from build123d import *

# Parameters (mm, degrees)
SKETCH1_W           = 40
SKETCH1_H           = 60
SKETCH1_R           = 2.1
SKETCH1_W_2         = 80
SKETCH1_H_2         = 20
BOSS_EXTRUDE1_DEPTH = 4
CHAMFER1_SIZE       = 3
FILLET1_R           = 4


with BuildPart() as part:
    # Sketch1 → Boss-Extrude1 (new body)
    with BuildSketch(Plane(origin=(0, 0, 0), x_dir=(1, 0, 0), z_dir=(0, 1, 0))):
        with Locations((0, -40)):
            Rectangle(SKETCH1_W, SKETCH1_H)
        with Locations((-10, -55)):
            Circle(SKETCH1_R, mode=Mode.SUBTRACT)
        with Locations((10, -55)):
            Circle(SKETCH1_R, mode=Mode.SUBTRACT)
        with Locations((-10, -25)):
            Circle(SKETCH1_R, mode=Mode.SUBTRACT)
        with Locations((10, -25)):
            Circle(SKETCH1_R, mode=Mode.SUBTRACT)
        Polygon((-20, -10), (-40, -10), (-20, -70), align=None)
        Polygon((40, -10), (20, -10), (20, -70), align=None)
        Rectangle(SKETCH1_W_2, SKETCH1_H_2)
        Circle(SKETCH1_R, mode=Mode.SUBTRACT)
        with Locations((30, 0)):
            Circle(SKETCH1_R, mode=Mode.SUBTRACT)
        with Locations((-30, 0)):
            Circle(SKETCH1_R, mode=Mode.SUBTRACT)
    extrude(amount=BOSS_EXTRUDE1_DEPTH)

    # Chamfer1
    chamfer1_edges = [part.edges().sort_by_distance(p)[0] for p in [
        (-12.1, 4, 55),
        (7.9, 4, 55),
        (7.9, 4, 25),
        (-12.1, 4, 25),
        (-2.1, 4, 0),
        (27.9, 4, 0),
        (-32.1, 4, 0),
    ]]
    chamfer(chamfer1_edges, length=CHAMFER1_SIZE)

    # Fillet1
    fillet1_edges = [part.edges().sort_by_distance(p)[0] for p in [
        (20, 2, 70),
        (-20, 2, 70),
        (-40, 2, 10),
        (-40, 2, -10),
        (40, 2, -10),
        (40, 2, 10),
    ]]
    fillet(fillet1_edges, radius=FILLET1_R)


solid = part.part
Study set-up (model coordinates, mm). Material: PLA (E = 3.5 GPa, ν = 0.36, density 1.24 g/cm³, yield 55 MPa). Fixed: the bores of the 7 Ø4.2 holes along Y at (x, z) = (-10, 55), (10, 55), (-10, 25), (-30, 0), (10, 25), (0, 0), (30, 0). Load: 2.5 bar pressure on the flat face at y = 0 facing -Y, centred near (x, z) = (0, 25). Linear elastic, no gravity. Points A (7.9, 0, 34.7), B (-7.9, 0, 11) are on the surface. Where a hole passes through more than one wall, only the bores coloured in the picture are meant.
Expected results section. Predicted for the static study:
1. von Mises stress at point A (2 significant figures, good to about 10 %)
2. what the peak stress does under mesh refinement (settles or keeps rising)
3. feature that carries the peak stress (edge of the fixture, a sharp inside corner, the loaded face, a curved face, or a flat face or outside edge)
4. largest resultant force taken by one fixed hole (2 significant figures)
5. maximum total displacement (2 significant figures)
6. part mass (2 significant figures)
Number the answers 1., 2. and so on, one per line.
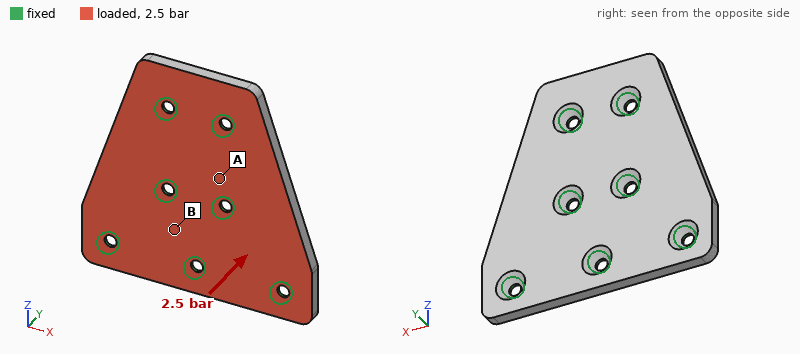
1. 6.9 MPa
2. keeps rising
3. edge of the fixture
4. 250 N
5. 0.45 mm
6. 25 g
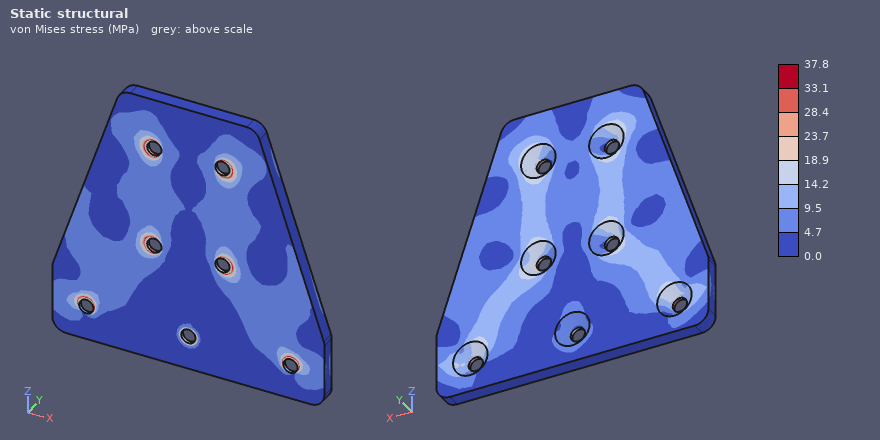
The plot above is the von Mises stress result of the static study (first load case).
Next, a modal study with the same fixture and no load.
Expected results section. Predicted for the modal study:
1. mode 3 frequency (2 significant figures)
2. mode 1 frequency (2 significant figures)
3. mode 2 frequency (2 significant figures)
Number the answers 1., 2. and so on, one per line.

1. 3100 Hz
2. 2100 Hz
3. 2100 Hz
